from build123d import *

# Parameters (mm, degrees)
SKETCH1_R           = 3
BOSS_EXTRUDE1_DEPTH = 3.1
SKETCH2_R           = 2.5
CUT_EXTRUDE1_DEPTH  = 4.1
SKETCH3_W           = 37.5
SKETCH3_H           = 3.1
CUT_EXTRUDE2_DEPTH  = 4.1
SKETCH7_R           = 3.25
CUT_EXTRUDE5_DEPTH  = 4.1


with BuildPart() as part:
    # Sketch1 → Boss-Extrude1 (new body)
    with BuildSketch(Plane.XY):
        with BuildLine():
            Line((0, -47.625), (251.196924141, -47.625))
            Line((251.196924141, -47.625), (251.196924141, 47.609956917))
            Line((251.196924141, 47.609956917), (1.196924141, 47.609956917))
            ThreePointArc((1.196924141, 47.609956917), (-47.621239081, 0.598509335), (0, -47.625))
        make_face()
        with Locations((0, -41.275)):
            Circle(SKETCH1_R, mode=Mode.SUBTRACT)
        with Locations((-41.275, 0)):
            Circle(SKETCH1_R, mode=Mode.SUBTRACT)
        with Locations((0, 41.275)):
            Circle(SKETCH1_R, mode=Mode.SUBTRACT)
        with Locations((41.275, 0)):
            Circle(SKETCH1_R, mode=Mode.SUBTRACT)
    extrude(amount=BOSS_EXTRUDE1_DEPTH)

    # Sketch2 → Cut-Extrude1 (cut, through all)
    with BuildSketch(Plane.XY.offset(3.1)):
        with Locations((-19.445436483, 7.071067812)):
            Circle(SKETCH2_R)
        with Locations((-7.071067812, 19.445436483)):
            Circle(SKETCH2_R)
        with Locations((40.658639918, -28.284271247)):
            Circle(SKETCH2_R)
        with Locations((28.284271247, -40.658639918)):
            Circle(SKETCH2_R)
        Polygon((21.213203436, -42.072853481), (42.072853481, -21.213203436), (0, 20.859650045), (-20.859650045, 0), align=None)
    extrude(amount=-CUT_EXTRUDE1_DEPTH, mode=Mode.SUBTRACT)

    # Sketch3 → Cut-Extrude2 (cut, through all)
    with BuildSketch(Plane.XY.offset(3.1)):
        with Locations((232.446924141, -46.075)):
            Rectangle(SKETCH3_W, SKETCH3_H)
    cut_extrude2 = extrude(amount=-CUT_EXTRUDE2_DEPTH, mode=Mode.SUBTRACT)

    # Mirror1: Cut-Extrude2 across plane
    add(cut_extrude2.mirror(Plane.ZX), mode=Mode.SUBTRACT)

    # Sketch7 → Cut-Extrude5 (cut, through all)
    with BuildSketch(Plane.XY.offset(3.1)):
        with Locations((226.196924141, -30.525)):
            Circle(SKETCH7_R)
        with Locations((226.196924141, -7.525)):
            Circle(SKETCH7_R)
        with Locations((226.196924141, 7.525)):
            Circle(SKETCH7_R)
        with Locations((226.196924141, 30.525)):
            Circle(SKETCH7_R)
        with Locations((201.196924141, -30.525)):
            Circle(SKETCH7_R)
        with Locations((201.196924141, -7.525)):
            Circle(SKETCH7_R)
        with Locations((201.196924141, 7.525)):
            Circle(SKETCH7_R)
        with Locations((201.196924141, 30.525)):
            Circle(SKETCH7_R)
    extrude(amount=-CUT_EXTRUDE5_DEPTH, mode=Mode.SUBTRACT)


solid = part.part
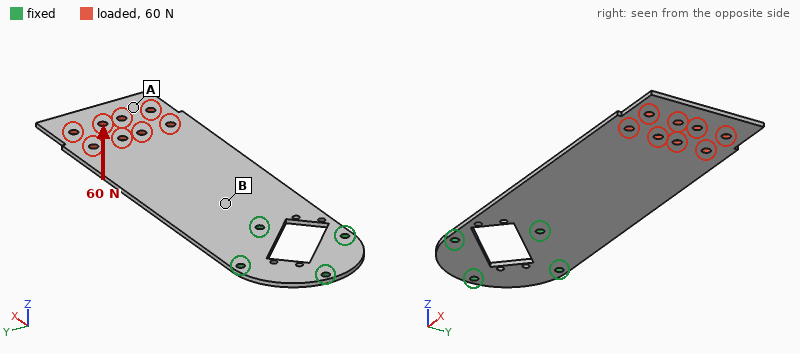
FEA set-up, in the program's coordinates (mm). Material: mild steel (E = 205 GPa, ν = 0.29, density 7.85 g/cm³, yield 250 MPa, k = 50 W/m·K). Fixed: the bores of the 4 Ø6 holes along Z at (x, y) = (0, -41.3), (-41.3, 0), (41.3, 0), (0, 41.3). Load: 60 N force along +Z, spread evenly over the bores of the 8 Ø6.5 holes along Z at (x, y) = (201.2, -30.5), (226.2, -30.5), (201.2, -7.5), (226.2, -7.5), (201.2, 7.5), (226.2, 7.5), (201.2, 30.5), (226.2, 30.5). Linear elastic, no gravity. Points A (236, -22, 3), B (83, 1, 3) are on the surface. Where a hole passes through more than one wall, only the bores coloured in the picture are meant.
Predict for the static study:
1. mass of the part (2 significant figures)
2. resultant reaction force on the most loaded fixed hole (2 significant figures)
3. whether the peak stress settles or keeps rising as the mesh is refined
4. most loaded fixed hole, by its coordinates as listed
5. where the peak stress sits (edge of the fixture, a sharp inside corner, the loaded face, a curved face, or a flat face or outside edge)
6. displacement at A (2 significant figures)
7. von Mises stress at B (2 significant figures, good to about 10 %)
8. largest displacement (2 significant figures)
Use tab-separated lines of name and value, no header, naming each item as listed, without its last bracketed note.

mass of the part	610 g
resultant reaction force on the most loaded fixed hole	180 N
whether the peak stress settles or keeps rising as the mesh is refined	keeps rising
most loaded fixed hole, by its coordinates as listed	(41.3, 0)
where the peak stress sits	edge of the fixture
displacement at A	2.7 mm
von Mises stress at B	45 MPa
largest displacement	3.0 mm
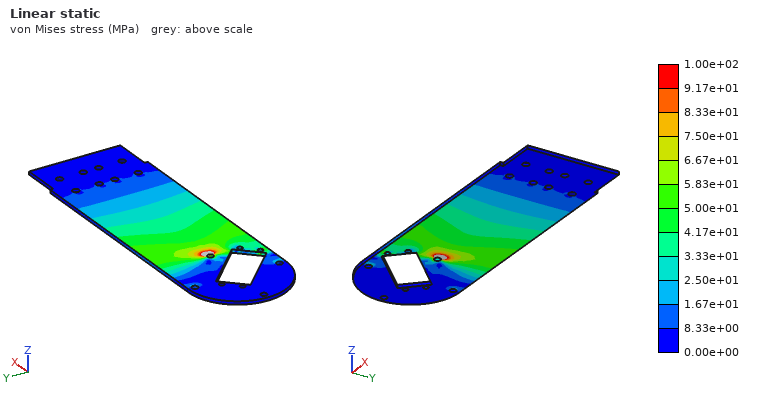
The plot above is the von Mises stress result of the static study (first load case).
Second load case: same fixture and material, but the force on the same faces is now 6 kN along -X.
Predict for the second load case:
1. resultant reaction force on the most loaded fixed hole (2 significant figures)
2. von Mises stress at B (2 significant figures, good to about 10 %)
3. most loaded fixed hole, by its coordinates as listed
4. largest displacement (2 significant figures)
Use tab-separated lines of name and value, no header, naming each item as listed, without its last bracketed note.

resultant reaction force on the most loaded fixed hole	4.1 kN
von Mises stress at B	26 MPa
most loaded fixed hole, by its coordinates as listed	(41.3, 0)
largest displacement	27 µm
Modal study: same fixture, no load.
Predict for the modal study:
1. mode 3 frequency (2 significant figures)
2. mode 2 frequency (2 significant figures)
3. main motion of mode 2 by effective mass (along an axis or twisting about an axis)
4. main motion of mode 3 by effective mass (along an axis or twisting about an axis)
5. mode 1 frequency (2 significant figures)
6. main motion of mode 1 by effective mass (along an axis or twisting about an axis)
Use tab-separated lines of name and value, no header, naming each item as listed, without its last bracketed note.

mode 3 frequency	340 Hz
mode 2 frequency	240 Hz
main motion of mode 2 by effective mass	twisting about X
main motion of mode 3 by effective mass	along Z
mode 1 frequency	58 Hz
main motion of mode 1 by effective mass	along Z
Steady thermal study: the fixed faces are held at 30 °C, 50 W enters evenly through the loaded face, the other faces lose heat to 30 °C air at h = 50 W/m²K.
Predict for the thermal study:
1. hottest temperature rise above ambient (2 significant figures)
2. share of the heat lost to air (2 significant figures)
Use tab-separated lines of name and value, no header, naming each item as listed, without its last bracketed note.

hottest temperature rise above ambient	75 K
share of the heat lost to air	99 %
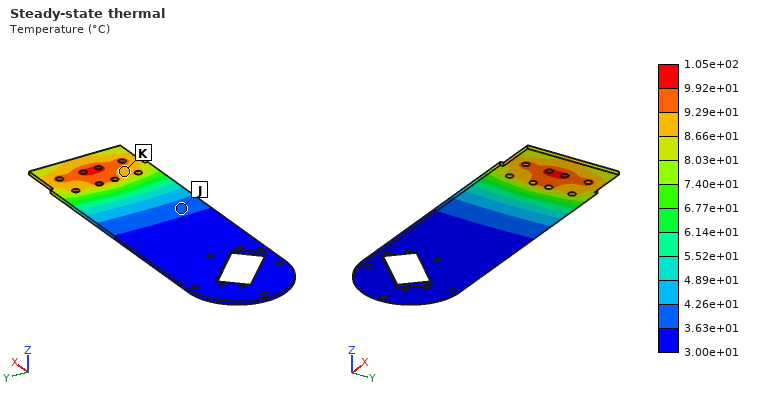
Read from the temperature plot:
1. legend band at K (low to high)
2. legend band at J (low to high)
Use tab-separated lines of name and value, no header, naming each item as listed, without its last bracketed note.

legend band at K	8.66e+01 to 9.29e+01 °C
legend band at J	3.63e+01 to 4.26e+01 °C
